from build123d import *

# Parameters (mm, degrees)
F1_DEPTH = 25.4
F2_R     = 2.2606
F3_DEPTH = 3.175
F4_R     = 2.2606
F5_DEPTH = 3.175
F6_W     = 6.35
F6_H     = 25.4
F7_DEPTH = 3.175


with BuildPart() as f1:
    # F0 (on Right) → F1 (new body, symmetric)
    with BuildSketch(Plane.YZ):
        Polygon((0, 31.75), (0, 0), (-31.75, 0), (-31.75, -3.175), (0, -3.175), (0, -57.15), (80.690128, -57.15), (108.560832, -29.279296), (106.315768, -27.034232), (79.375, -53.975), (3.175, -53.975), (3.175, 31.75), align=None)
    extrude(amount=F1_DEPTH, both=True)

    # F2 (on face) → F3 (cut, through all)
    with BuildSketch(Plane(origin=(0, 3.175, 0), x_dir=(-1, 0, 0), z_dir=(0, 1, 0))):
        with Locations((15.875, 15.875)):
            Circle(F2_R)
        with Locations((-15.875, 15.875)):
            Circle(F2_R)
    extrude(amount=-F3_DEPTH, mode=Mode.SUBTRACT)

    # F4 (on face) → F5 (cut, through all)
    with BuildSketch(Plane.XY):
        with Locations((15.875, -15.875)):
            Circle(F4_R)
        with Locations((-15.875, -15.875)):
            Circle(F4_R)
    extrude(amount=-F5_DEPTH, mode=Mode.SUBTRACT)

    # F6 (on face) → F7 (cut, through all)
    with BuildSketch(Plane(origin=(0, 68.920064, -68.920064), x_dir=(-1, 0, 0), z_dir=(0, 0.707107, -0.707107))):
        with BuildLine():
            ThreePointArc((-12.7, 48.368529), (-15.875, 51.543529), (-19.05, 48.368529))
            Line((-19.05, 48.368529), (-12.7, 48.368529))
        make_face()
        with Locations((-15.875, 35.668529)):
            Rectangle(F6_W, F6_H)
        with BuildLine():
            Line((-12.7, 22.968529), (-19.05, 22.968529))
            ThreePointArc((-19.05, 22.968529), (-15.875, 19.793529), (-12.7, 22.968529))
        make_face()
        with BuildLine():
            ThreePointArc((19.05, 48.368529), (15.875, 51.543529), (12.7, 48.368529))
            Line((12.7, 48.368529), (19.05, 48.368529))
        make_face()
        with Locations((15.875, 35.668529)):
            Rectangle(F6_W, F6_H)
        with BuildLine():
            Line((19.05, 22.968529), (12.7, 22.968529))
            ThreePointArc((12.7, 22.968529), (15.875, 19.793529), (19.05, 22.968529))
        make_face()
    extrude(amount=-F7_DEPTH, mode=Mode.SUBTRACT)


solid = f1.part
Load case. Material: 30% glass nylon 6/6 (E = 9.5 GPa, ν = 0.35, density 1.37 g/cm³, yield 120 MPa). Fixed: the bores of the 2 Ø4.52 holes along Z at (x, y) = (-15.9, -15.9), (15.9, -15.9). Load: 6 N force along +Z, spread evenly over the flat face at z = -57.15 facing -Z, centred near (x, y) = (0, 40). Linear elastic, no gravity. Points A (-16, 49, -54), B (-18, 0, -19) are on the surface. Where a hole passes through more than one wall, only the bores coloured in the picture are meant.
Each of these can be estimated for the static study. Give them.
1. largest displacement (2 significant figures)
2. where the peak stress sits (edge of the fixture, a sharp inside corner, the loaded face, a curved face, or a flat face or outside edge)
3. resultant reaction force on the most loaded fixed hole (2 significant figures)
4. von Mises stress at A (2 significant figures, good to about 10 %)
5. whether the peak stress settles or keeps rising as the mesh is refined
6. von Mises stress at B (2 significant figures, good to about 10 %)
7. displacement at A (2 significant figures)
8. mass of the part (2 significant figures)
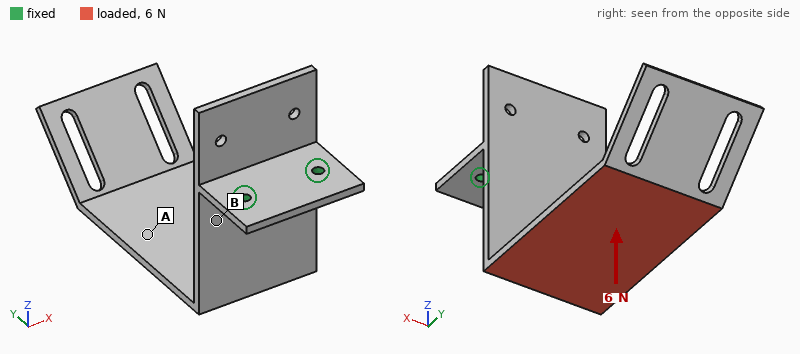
1.7 mm
edge of the fixture
3.3 N
0.44 MPa
keeps rising
2.5 MPa
0.83 mm
50 g
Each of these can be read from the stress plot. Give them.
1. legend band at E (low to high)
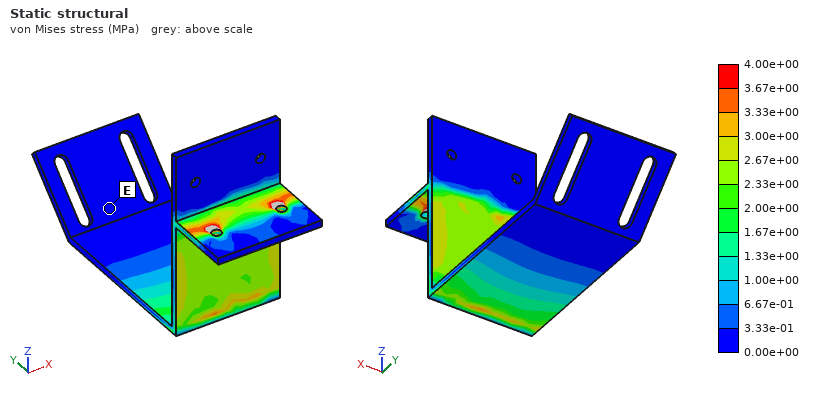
0.00e+00 to 3.33e-01 MPa
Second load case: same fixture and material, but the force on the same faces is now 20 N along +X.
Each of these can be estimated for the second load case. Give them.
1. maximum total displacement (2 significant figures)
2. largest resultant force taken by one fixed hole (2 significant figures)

1.7 mm
47 N
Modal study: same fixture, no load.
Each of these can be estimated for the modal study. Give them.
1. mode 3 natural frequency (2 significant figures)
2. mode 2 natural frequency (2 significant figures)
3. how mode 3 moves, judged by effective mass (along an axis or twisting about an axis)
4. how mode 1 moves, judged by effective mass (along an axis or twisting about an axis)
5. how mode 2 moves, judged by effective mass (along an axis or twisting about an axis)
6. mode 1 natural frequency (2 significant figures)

180 Hz
110 Hz
along Y
along Z
along X
57 Hz
